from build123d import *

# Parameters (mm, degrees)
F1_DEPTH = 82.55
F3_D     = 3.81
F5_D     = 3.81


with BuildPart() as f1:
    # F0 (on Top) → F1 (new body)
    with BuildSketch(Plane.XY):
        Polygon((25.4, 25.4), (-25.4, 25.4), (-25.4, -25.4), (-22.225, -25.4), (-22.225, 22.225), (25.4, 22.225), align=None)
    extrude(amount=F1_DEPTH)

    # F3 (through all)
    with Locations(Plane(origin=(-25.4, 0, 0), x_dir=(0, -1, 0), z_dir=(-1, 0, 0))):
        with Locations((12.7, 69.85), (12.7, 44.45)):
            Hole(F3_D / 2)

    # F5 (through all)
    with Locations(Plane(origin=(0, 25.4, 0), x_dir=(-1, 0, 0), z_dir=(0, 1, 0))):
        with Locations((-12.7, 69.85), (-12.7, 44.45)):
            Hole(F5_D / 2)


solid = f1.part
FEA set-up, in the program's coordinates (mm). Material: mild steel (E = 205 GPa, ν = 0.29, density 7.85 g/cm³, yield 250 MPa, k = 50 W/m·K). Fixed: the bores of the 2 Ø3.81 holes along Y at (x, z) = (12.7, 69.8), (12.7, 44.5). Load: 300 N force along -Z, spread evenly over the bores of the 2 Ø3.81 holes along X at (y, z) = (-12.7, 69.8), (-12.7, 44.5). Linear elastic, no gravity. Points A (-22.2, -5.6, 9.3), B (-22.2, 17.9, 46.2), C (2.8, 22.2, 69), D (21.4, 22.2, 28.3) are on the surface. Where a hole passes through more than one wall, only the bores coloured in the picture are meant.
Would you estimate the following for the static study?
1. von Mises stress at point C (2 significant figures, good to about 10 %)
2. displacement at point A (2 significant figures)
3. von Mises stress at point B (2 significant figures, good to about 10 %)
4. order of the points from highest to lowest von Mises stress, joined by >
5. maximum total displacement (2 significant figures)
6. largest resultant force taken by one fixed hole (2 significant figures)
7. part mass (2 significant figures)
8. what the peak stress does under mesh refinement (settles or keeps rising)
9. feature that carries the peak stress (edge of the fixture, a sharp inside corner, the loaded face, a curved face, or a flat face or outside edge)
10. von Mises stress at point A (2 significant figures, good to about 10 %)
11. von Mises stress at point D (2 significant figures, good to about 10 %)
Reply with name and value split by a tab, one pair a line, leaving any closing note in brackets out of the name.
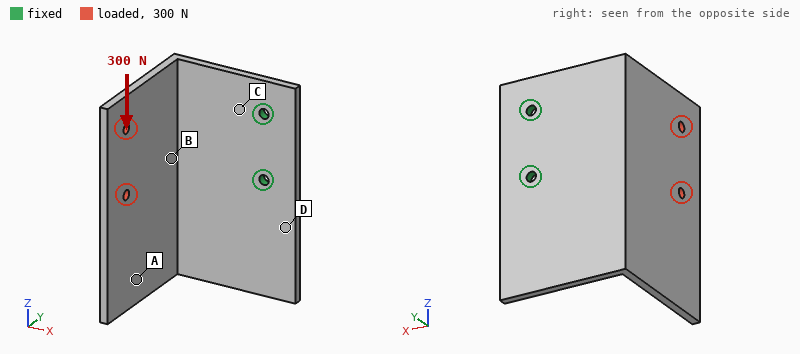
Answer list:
von Mises stress at point C	61 MPa
displacement at point A	0.23 mm
von Mises stress at point B	28 MPa
order of the points from highest to lowest von Mises stress, joined by >	C > D > B > A
maximum total displacement	0.32 mm
largest resultant force taken by one fixed hole	520 N
part mass	200 g
what the peak stress does under mesh refinement	keeps rising
feature that carries the peak stress	edge of the fixture
von Mises stress at point A	10 MPa
von Mises stress at point D	45 MPa
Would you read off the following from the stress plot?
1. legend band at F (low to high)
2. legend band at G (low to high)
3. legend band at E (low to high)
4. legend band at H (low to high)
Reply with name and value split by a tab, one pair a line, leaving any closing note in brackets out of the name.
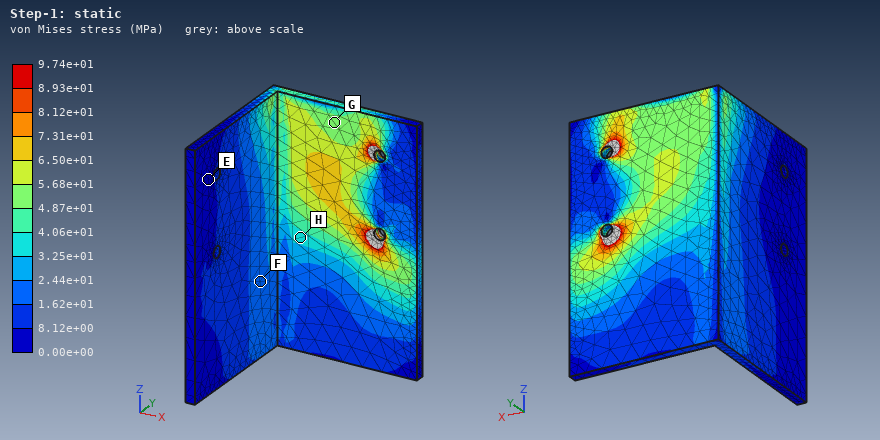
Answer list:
legend band at F	1.62e+01 to 2.44e+01 MPa
legend band at G	4.87e+01 to 5.68e+01 MPa
legend band at E	0.00e+00 to 8.12e+00 MPa
legend band at H	3.25e+01 to 4.06e+01 MPa
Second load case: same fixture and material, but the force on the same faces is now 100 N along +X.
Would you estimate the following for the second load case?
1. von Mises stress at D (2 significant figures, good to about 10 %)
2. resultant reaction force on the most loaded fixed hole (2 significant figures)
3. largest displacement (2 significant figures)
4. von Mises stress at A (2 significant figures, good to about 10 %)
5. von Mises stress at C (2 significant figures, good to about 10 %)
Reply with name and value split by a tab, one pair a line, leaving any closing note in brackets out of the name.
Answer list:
von Mises stress at D	15 MPa
resultant reaction force on the most loaded fixed hole	51 N
largest displacement	0.24 mm
von Mises stress at A	8.3 MPa
von Mises stress at C	31 MPa
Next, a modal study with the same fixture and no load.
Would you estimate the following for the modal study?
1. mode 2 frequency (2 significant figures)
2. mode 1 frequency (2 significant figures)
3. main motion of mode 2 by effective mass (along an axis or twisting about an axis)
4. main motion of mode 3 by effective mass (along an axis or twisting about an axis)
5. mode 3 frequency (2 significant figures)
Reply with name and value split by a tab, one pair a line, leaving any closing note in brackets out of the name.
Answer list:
mode 2 frequency	640 Hz
mode 1 frequency	420 Hz
main motion of mode 2 by effective mass	along Z
main motion of mode 3 by effective mass	along Y
mode 3 frequency	1200 Hz
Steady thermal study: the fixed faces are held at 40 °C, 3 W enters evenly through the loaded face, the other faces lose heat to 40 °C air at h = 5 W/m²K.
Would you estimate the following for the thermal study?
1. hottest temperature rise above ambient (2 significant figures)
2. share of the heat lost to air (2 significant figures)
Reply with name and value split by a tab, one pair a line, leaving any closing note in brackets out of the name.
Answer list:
hottest temperature rise above ambient	20 K
share of the heat lost to air	25 %
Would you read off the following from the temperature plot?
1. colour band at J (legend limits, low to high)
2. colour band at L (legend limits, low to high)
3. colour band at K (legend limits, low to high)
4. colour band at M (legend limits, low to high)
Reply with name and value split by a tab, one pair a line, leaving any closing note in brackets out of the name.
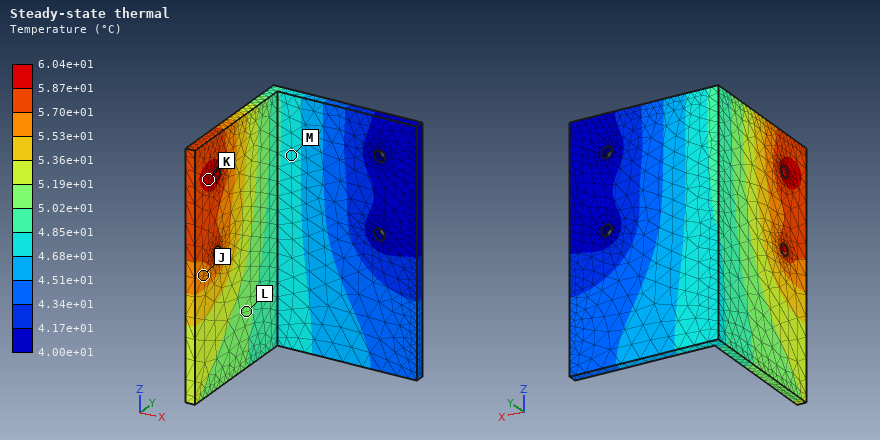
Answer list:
colour band at J	5.53e+01 to 5.70e+01 °C
colour band at L	5.02e+01 to 5.19e+01 °C
colour band at K	5.87e+01 to 6.04e+01 °C
colour band at M	4.68e+01 to 4.85e+01 °C
